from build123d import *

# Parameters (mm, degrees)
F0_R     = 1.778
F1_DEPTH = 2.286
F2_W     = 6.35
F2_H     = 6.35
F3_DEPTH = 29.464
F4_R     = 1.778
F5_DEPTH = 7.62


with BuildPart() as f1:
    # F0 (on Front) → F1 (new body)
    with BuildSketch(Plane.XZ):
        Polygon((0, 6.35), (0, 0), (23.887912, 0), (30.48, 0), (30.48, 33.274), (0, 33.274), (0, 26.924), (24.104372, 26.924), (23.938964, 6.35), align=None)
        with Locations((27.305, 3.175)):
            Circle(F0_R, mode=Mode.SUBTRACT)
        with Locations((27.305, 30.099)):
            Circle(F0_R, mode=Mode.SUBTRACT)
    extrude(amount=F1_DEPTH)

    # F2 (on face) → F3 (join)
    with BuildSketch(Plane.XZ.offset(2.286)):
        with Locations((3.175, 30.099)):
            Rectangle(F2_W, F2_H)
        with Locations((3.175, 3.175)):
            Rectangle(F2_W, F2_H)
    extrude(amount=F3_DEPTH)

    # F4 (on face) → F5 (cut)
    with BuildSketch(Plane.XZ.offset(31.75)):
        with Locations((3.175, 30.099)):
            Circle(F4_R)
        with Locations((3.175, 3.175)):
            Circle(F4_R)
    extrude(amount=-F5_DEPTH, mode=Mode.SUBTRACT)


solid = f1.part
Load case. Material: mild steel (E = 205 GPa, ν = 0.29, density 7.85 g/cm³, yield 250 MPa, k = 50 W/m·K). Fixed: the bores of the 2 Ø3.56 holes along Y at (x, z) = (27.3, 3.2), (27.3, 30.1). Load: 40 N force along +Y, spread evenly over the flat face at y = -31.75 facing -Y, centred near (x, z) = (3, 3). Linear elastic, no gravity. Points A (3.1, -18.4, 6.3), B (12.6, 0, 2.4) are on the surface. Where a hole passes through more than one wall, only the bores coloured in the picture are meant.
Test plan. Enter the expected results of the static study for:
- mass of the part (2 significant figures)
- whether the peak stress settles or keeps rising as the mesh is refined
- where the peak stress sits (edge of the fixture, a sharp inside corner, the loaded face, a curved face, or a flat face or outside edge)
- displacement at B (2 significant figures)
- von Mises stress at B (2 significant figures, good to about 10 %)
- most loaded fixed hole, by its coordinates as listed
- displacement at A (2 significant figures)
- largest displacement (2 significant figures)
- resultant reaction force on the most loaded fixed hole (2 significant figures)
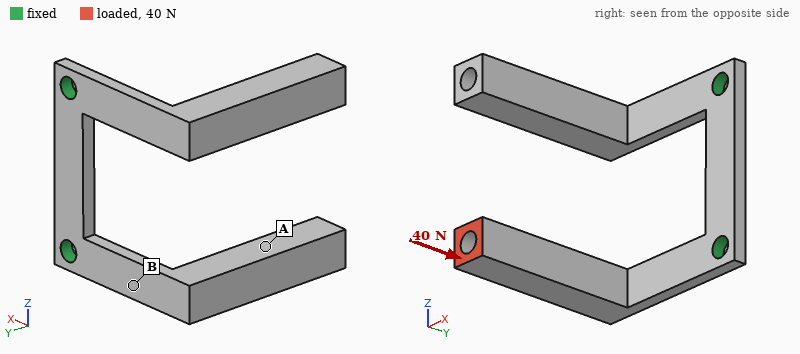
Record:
26 g
keeps rising
edge of the fixture
0.050 mm
68 MPa
(27.3, 3.2)
0.18 mm
0.28 mm
42 N
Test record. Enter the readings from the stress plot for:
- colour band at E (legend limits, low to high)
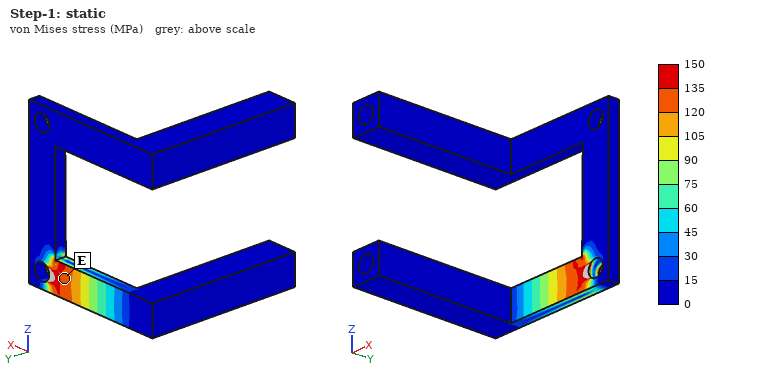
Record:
120 to 135 MPa
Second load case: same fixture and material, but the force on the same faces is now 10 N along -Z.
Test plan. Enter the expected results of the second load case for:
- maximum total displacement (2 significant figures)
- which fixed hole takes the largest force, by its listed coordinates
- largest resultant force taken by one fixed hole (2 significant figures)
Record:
0.12 mm
(27.3, 3.2)
7.5 N
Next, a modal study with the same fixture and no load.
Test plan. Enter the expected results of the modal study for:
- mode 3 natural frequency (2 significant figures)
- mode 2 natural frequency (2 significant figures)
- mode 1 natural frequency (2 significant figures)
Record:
840 Hz
610 Hz
610 Hz
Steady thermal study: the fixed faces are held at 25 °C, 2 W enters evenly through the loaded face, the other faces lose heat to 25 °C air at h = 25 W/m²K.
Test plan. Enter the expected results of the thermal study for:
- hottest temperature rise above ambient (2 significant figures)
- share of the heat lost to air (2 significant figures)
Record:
54 K
52 %
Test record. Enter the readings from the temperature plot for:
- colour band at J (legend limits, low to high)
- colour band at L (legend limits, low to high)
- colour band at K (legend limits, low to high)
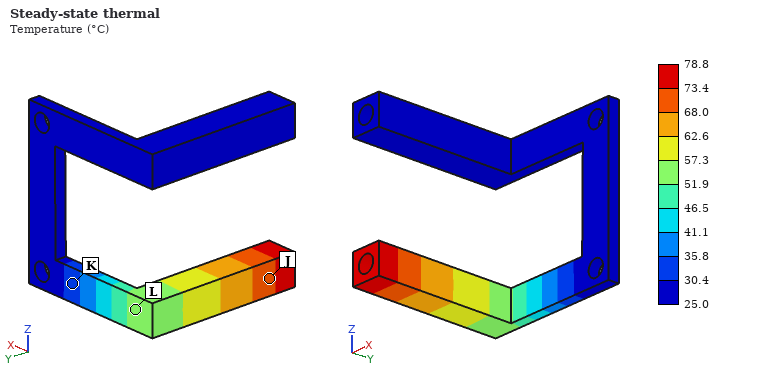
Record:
68.0 to 73.4 °C
51.9 to 57.3 °C
30.4 to 35.8 °C
